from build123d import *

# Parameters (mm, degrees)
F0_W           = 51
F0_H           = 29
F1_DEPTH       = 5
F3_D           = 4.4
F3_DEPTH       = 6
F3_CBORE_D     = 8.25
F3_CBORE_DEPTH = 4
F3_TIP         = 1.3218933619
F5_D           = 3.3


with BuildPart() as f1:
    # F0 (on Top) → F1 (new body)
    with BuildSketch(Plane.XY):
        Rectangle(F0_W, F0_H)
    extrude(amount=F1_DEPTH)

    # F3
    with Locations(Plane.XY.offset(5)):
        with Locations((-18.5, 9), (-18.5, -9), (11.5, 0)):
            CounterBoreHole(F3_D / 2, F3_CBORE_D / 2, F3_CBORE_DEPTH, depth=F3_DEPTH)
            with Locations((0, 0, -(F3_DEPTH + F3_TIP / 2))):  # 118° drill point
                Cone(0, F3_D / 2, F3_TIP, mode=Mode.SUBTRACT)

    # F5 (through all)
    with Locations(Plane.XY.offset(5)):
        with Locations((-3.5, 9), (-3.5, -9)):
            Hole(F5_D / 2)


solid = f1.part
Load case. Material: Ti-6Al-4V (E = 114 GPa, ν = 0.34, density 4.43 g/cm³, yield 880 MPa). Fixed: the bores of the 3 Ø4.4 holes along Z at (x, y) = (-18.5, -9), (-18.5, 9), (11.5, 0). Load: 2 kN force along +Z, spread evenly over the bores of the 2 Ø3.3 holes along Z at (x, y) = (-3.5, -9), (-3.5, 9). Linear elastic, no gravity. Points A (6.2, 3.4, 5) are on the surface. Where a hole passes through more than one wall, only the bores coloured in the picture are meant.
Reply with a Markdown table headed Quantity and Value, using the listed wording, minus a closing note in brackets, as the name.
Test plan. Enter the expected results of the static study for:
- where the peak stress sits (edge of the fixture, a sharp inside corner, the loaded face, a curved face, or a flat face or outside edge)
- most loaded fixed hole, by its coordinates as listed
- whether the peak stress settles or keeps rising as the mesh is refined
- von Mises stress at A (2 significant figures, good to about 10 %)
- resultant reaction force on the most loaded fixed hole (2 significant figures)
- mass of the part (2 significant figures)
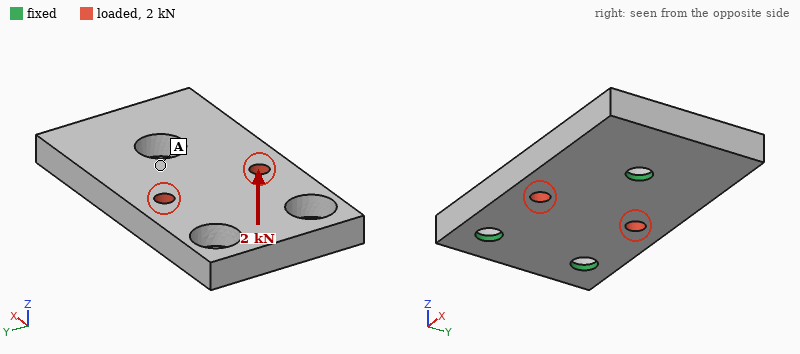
| Quantity | Value |
|---|---|
| where the peak stress sits | edge of the fixture |
| most loaded fixed hole, by its coordinates as listed | (11.5, 0) |
| whether the peak stress settles or keeps rising as the mesh is refined | keeps rising |
| von Mises stress at A | 48 MPa |
| resultant reaction force on the most loaded fixed hole | 1.7 kN |
| mass of the part | 29 g |
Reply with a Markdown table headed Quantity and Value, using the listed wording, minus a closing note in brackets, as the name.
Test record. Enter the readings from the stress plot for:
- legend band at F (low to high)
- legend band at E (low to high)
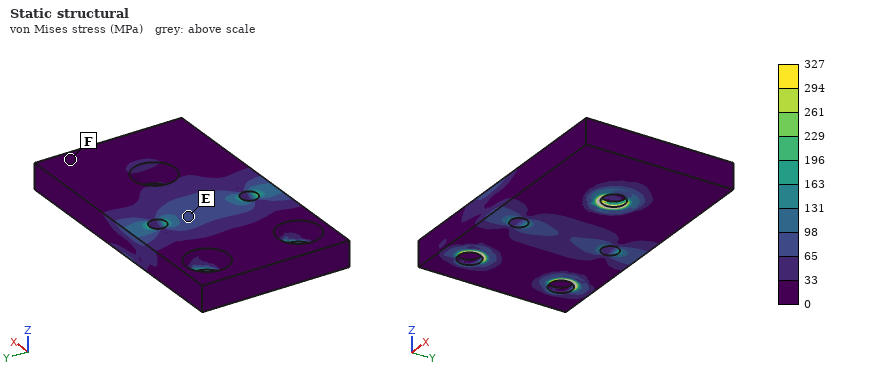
| Quantity | Value |
|---|---|
| legend band at F | 0 to 33 MPa |
| legend band at E | 65 to 98 MPa |
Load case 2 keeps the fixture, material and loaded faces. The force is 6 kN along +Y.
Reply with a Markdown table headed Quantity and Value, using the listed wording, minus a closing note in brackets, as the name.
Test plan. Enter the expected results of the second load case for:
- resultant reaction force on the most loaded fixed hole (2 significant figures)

| Quantity | Value |
|---|---|
| resultant reaction force on the most loaded fixed hole | 2.4 kN |
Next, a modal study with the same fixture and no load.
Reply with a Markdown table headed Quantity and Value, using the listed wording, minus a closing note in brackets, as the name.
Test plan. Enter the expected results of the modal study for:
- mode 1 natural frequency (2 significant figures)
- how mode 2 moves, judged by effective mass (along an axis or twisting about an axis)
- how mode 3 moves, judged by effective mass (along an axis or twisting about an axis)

| Quantity | Value |
|---|---|
| mode 1 natural frequency | 6900 Hz |
| how mode 2 moves, judged by effective mass | along Z |
| how mode 3 moves, judged by effective mass | along Z |
